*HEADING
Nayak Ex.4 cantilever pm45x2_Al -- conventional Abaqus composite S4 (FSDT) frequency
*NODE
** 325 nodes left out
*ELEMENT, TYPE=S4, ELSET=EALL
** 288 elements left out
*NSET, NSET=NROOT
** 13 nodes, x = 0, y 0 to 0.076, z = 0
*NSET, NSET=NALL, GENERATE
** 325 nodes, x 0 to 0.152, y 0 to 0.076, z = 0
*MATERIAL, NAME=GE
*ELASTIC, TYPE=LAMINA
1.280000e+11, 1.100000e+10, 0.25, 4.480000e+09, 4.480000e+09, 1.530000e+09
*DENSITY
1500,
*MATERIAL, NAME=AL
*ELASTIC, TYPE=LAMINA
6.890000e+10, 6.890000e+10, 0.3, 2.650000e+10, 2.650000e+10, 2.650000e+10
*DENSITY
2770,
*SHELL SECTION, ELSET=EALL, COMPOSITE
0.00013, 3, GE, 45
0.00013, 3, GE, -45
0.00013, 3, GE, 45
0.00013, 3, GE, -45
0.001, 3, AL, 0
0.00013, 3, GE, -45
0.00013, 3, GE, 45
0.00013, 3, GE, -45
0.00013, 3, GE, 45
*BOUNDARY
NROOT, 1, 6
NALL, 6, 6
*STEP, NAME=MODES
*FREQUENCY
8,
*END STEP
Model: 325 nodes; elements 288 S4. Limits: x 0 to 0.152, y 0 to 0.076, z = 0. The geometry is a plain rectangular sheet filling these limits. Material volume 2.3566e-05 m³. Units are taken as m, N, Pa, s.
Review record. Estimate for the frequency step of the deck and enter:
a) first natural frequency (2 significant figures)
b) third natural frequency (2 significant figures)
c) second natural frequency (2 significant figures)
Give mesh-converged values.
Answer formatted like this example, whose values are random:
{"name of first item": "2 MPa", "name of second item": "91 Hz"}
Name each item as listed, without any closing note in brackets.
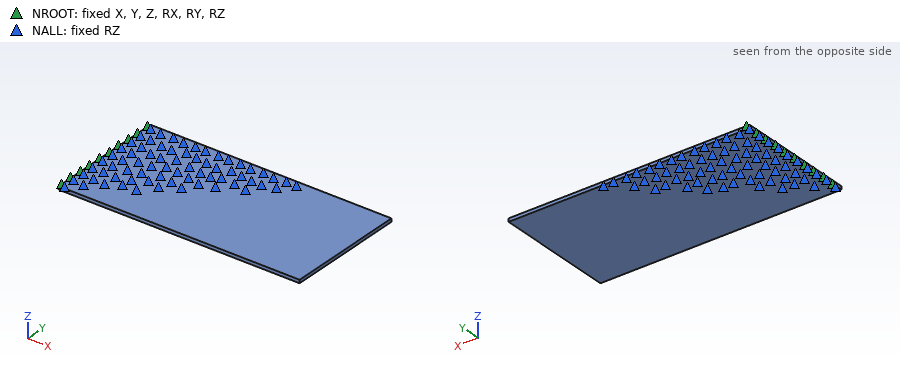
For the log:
{"first natural frequency": "58 Hz", "third natural frequency": "370 Hz", "second natural frequency": "350 Hz"}
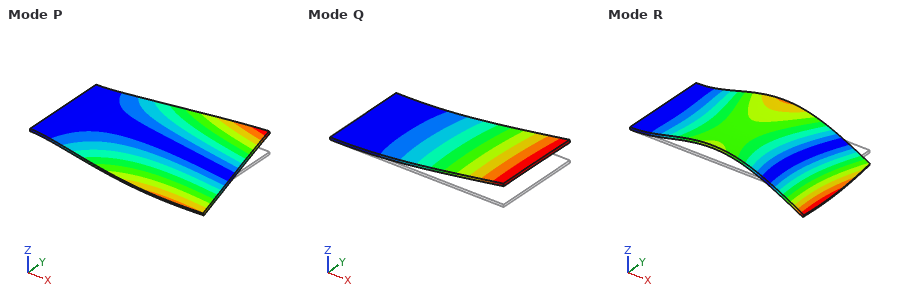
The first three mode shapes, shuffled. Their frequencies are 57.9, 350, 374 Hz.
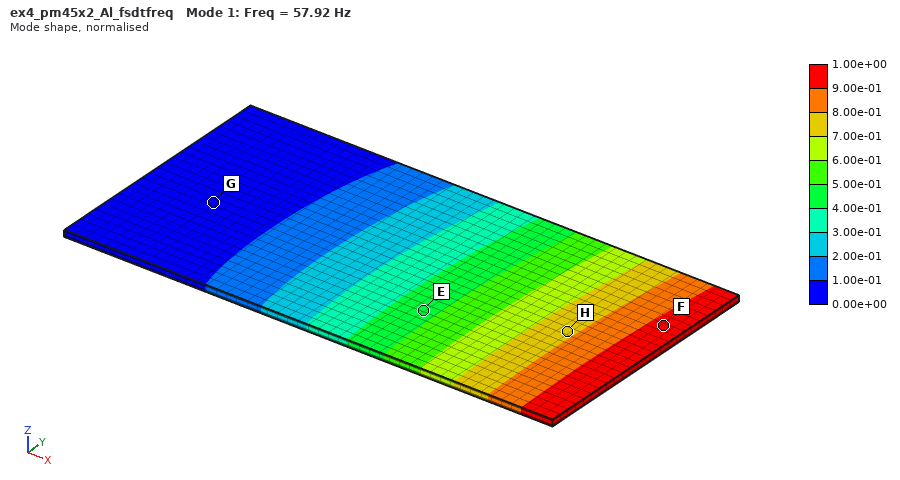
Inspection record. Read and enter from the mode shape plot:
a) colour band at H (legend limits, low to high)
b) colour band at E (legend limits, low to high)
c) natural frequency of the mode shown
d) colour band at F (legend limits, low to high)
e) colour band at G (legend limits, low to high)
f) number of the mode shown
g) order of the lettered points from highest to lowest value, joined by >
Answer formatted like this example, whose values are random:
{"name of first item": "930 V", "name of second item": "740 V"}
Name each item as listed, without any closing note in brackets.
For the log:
{"colour band at H": "7.00e-01 to 8.00e-01", "colour band at E": "4.00e-01 to 5.00e-01", "natural frequency of the mode shown": "57.92 Hz", "colour band at F": "9.00e-01 to 1.00e+00", "colour band at G": "0.00e+00 to 1.00e-01", "number of the mode shown": "1", "order of the lettered points from highest to lowest value, joined by >": "F > H > E > G"}
